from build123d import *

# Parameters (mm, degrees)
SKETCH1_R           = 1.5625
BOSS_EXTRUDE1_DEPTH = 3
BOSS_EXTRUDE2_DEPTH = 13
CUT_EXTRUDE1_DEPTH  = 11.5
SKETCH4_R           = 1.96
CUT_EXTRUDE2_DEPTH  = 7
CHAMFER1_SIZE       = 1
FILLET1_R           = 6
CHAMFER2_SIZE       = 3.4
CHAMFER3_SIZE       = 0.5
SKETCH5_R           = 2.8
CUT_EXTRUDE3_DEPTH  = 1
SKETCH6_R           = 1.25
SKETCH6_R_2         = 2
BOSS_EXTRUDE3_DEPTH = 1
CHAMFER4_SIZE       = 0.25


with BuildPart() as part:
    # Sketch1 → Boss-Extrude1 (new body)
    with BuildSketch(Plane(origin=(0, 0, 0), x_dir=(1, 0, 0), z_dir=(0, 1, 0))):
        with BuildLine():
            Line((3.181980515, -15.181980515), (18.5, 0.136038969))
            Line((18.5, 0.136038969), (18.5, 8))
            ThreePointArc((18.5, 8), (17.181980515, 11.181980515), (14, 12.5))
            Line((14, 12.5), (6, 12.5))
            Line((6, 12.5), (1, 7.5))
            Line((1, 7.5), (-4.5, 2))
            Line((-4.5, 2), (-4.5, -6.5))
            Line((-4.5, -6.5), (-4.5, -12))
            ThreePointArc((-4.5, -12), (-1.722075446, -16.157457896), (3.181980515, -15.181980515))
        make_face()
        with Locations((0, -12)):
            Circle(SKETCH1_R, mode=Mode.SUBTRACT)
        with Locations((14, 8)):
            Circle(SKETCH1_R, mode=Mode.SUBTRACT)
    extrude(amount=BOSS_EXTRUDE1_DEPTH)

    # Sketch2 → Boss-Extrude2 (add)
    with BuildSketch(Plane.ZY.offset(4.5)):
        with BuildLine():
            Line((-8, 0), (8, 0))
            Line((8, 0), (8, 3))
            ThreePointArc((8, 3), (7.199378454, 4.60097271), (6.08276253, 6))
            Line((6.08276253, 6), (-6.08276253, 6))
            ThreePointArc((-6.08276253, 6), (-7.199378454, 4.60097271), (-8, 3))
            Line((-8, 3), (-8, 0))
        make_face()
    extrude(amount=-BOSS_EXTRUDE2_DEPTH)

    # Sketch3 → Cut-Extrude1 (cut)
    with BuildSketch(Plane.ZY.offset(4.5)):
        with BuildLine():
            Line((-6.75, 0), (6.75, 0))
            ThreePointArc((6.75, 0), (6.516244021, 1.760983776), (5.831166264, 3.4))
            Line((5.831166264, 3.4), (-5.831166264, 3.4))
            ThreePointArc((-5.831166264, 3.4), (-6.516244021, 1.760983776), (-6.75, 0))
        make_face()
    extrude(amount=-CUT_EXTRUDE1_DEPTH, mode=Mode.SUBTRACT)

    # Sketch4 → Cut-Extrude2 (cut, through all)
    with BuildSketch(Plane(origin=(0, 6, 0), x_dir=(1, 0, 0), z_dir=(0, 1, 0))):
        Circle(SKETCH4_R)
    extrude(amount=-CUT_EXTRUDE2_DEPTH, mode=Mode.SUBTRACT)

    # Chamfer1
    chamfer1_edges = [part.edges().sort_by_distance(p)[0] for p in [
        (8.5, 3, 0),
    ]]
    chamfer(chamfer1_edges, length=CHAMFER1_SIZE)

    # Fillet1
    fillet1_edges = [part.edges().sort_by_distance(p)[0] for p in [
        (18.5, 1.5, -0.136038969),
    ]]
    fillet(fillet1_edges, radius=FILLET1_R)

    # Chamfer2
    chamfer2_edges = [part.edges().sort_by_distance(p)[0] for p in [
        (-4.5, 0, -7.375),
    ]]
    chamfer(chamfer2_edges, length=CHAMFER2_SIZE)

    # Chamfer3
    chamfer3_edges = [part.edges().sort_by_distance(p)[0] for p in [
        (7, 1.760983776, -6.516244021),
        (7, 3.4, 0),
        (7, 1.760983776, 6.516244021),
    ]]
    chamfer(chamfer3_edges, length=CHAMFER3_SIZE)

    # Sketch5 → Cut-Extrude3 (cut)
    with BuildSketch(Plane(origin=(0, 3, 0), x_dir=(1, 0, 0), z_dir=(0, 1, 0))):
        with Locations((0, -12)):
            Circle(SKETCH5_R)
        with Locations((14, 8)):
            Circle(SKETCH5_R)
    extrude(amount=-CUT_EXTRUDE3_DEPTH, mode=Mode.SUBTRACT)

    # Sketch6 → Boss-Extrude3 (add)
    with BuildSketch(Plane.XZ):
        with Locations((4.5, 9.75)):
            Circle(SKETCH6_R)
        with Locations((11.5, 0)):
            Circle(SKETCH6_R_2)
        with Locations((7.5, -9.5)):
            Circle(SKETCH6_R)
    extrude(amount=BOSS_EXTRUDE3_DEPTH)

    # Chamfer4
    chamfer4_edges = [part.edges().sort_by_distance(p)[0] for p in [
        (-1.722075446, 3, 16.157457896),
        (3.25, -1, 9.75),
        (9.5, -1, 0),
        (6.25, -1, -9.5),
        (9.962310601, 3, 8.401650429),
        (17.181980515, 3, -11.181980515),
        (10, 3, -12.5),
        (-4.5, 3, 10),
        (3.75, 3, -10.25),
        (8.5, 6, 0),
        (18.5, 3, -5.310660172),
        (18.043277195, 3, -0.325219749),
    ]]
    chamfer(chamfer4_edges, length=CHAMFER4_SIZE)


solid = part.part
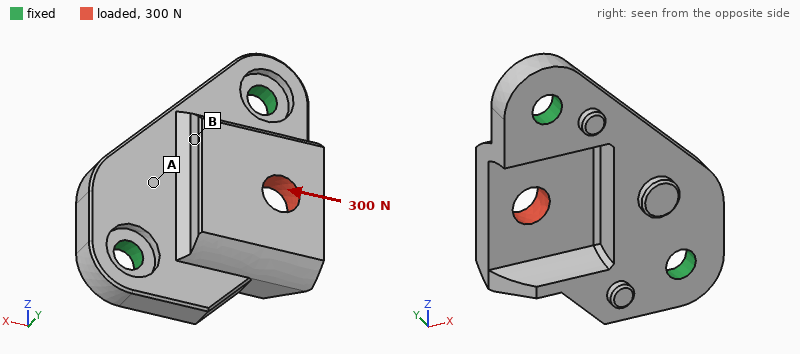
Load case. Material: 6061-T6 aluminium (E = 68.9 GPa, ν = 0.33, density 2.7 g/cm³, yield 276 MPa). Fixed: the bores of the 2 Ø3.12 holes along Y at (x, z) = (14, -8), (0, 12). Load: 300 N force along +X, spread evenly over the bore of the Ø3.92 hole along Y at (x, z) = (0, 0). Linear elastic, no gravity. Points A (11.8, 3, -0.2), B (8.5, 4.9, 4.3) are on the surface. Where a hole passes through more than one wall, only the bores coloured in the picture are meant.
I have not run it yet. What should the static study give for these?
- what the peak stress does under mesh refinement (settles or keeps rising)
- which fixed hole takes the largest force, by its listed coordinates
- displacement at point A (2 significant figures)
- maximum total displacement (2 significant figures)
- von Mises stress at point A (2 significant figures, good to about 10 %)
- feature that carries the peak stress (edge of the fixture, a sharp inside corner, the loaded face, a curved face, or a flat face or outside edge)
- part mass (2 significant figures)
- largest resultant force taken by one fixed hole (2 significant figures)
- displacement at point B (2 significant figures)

keeps rising
(0, 12)
5.2 µm
27 µm
14 MPa
edge of the fixture
3.8 g
170 N
8.5 µm
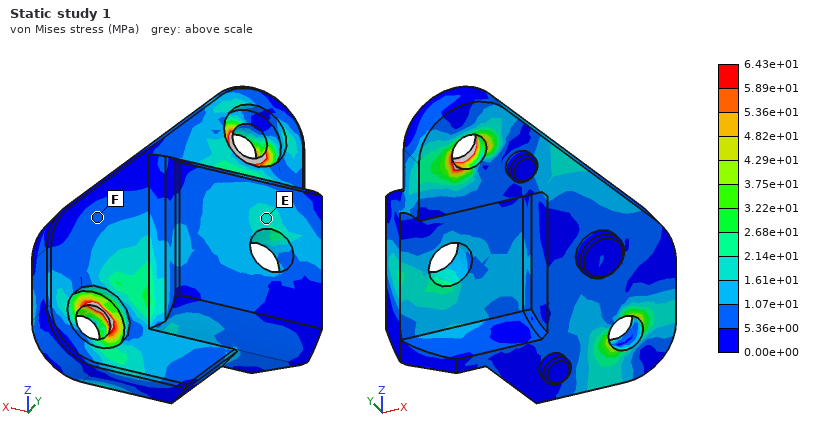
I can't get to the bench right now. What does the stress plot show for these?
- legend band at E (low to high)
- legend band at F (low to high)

1.61e+01 to 2.14e+01 MPa
5.36e+00 to 1.07e+01 MPa
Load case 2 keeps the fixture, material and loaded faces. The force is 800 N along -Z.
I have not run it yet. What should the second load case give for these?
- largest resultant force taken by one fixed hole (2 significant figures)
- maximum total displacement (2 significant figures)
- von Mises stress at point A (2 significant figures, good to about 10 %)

490 N
38 µm
21 MPa
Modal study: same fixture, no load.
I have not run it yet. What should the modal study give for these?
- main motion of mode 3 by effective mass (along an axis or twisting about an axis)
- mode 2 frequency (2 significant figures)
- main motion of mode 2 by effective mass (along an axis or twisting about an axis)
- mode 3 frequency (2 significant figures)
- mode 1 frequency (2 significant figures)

along Z
22 kHz
along Y
28 kHz
11 kHz
